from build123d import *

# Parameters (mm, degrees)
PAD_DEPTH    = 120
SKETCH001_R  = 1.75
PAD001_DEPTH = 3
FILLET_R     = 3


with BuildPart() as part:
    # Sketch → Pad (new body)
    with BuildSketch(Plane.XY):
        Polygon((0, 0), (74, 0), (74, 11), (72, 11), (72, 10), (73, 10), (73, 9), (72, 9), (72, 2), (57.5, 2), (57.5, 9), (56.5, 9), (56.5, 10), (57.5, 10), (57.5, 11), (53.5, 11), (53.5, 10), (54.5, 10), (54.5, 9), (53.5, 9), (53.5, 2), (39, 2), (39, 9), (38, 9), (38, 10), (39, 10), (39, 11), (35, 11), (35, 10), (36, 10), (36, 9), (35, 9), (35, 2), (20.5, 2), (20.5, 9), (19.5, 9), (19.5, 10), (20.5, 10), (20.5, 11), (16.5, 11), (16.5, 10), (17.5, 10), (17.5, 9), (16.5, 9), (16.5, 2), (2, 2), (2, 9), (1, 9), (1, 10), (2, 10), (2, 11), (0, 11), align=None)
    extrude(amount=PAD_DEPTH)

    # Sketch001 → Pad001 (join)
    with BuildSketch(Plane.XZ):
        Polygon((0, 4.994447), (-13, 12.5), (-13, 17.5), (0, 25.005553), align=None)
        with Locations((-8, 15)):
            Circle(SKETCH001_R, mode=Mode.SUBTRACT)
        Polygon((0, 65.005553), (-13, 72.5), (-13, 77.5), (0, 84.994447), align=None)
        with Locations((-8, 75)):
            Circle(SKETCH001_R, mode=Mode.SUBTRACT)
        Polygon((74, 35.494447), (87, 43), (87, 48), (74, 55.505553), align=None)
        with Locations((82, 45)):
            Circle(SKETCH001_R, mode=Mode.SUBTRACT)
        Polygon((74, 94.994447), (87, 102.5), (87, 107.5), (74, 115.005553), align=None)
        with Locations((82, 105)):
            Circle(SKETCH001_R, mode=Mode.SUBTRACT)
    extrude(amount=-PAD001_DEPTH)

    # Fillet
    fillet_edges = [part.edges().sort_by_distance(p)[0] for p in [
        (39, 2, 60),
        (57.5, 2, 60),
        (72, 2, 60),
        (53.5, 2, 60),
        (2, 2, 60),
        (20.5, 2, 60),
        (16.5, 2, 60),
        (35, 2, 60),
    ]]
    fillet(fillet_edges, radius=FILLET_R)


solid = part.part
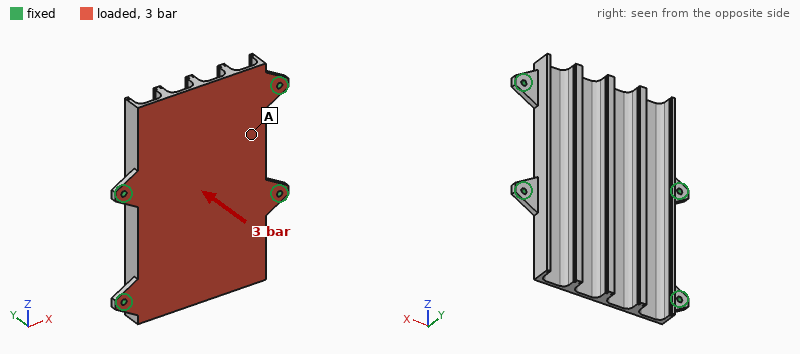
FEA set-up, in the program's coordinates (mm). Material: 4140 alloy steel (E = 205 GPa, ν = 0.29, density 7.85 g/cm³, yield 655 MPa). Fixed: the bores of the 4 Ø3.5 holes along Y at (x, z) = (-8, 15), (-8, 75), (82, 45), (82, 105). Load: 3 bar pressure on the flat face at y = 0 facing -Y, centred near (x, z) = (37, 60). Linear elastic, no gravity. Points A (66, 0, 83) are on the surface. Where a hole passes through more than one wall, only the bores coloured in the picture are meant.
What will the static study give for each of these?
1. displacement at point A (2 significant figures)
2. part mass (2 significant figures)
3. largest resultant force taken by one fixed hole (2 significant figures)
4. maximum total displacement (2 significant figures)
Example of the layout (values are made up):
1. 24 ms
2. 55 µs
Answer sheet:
1. 0.12 mm
2. 300 g
3. 1.5 kN
4. 0.34 mm
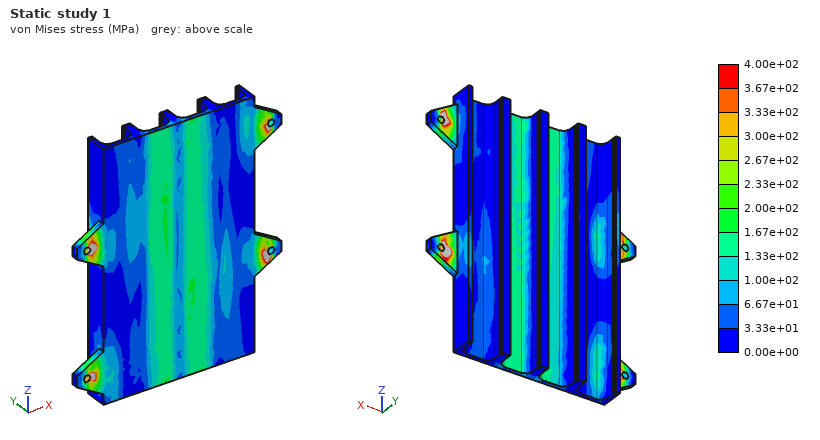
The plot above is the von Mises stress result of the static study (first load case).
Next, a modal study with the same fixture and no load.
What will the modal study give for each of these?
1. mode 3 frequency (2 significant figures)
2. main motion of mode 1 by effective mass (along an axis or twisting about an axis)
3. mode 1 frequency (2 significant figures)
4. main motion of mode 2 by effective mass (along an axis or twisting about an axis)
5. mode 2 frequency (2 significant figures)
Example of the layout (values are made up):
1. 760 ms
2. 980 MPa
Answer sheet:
1. 2600 Hz
2. along Y
3. 960 Hz
4. twisting about X
5. 1200 Hz
